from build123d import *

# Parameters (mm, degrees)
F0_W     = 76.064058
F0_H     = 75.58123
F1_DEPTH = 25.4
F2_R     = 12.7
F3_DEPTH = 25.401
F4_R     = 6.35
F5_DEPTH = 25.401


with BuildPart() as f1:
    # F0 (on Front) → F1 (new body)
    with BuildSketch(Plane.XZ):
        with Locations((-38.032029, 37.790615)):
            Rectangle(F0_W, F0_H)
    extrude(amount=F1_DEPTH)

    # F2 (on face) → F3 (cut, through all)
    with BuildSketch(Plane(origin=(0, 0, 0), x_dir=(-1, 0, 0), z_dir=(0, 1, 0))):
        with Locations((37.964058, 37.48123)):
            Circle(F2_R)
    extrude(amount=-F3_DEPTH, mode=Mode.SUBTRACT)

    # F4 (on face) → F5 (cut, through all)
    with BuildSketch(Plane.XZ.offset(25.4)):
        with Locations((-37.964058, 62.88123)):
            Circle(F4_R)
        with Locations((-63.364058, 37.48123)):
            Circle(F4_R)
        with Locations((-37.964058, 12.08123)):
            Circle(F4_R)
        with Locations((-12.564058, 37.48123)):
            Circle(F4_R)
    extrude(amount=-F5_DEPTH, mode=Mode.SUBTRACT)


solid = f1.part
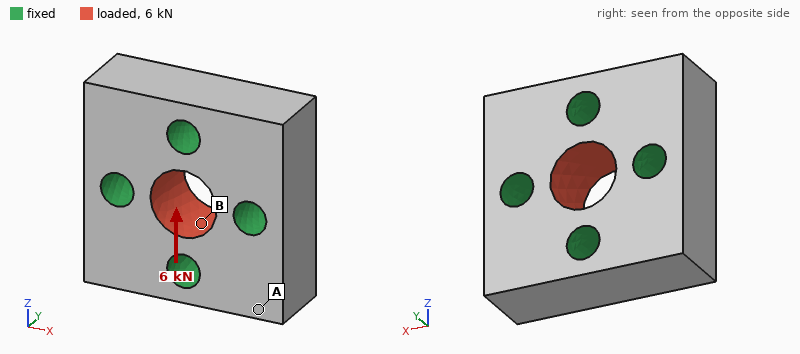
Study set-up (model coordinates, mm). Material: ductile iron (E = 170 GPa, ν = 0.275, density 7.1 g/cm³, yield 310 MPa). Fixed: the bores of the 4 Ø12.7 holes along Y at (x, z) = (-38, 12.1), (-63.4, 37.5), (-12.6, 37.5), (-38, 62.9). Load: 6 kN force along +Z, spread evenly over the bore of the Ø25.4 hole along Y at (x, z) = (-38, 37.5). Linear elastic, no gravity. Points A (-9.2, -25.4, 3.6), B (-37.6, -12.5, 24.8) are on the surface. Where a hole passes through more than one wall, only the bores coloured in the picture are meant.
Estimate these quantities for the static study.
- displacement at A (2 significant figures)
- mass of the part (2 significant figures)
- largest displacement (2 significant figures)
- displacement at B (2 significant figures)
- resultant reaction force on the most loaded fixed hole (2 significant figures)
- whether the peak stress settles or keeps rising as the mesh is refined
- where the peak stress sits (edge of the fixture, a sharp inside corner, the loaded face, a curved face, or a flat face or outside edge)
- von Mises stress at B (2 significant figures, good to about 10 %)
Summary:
0.063 µm
850 g
0.28 µm
0.12 µm
1.8 kN
keeps rising
edge of the fixture
3.8 MPa
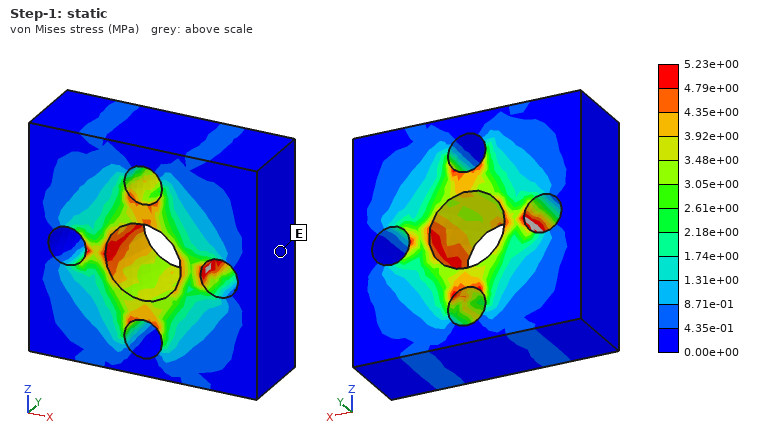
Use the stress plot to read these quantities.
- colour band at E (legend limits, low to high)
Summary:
0.00e+00 to 4.35e-01 MPa
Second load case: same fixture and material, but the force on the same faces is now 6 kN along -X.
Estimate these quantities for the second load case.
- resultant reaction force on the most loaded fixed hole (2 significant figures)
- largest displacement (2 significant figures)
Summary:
1.8 kN
0.28 µm
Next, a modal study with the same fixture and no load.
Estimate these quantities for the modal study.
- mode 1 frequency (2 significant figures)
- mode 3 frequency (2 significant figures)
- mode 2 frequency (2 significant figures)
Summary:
20 kHz
20 kHz
20 kHz
